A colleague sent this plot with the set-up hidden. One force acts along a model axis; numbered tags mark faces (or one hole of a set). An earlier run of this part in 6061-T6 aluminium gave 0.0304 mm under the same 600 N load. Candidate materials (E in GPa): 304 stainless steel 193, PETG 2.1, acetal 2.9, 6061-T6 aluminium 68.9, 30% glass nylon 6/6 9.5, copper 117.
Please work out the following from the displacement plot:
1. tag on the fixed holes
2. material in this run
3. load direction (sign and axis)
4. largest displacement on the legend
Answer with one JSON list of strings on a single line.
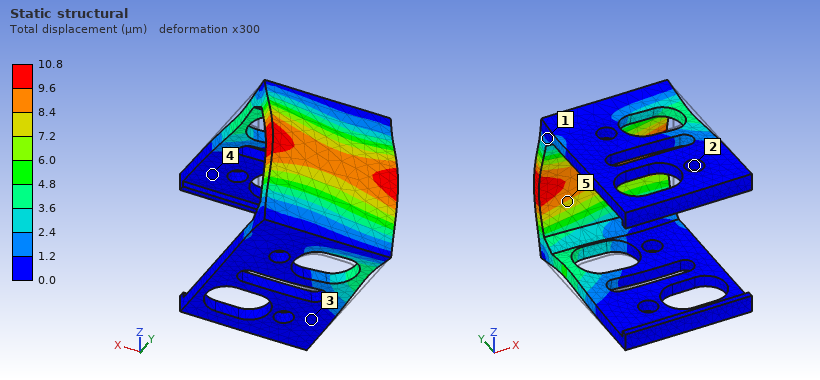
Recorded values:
["2", "304 stainless steel", "+Y", "10.8 µm"]
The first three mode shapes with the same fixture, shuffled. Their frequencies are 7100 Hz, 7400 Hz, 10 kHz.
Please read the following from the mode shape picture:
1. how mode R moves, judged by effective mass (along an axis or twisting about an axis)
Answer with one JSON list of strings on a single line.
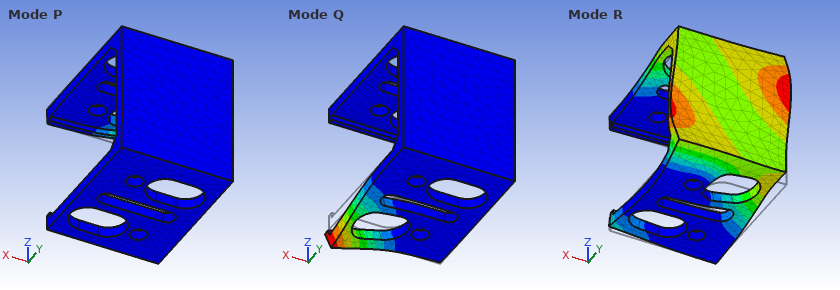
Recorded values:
["along Z"]
